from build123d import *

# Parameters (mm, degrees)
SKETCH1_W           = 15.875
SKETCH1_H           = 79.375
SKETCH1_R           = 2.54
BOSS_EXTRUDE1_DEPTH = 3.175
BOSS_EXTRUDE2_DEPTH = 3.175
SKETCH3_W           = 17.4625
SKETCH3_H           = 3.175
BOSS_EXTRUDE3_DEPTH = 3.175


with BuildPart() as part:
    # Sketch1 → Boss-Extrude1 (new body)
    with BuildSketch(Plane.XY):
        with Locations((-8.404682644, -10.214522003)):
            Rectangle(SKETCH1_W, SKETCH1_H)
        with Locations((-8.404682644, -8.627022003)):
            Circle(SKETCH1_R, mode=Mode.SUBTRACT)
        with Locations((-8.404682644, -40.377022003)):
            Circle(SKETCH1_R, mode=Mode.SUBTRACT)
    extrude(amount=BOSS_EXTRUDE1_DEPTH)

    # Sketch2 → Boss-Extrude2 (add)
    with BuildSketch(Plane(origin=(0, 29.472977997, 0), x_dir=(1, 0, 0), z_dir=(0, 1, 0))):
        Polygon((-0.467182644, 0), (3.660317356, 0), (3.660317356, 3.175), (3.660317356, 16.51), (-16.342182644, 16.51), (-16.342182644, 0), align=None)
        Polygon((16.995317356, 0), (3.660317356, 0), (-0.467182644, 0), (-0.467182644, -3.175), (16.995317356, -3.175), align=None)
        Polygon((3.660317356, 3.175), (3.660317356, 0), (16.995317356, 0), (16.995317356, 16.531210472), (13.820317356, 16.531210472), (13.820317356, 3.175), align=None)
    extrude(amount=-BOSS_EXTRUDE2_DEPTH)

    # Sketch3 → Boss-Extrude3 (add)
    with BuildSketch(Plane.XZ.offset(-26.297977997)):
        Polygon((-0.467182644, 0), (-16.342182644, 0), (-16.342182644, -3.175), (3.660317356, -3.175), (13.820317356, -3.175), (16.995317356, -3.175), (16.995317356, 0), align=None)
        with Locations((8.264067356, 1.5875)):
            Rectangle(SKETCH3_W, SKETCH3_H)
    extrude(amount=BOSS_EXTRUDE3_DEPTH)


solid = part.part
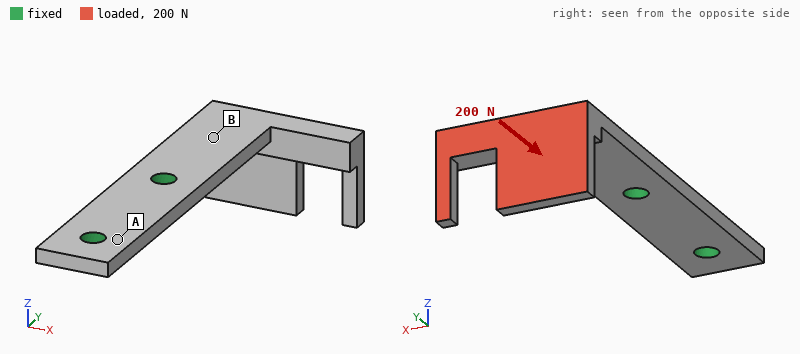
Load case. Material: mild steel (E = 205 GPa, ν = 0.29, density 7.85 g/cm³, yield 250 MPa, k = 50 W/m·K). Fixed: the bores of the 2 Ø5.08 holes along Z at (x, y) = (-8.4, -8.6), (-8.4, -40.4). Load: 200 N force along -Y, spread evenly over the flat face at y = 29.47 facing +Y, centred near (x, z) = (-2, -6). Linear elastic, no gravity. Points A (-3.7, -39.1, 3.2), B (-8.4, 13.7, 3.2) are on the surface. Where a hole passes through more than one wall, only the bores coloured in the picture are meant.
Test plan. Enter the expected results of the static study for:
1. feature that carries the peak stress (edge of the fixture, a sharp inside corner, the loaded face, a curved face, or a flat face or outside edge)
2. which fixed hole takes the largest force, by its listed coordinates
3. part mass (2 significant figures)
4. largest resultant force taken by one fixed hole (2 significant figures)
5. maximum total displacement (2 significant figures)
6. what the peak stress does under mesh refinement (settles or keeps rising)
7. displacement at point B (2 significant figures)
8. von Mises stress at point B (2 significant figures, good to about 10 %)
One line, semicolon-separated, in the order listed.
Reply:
edge of the fixture; (-8.4, -8.6); 46 g; 190 N; 0.16 mm; keeps rising; 0.038 mm; 50 MPa
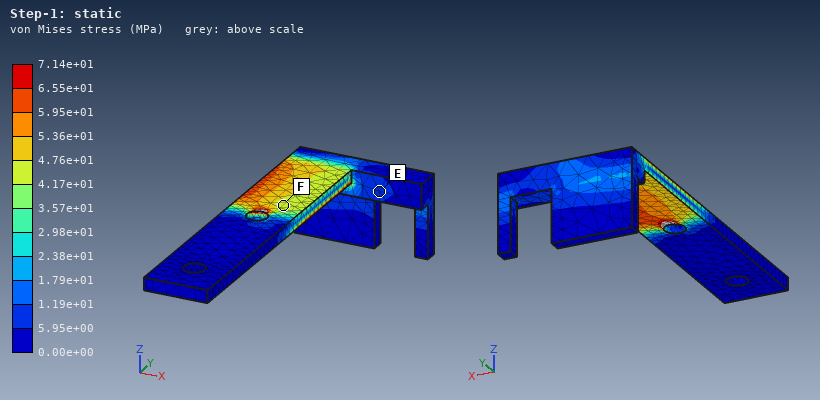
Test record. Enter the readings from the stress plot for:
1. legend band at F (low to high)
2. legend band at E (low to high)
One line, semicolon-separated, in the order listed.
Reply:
4.17e+01 to 4.76e+01 MPa; 5.95e+00 to 1.19e+01 MPa
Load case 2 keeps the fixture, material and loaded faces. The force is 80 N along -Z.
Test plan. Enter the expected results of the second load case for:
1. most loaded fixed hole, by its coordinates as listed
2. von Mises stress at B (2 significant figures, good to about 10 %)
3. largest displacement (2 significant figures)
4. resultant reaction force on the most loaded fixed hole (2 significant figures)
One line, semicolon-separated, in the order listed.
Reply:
(-8.4, -8.6); 49 MPa; 0.22 mm; 82 N
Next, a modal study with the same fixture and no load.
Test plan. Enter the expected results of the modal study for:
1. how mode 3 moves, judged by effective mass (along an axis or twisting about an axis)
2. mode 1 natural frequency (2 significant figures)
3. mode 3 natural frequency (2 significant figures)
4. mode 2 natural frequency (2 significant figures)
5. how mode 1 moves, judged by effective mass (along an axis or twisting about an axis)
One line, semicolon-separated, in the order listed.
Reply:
along X; 830 Hz; 3500 Hz; 1800 Hz; along Z
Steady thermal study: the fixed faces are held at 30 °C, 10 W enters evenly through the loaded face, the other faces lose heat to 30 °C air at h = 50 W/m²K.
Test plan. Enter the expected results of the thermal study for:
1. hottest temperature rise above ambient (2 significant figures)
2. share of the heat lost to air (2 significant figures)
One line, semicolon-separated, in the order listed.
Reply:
78 K; 58 %
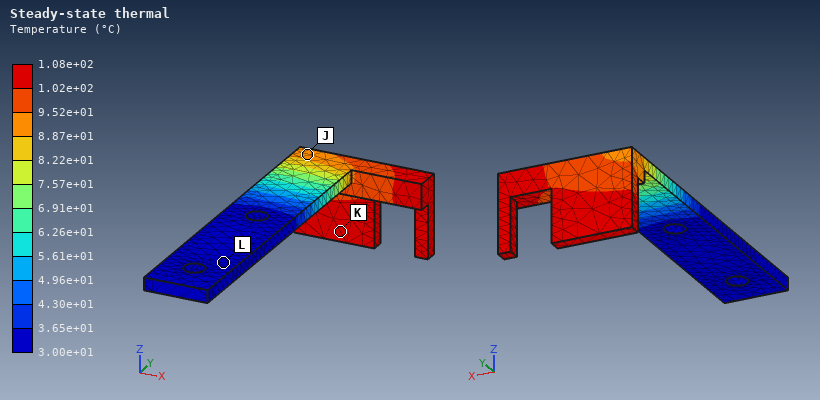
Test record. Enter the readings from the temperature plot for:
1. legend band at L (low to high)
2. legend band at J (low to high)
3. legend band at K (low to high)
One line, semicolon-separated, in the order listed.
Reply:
3.00e+01 to 3.65e+01 °C; 8.87e+01 to 9.52e+01 °C; 1.02e+02 to 1.08e+02 °C
